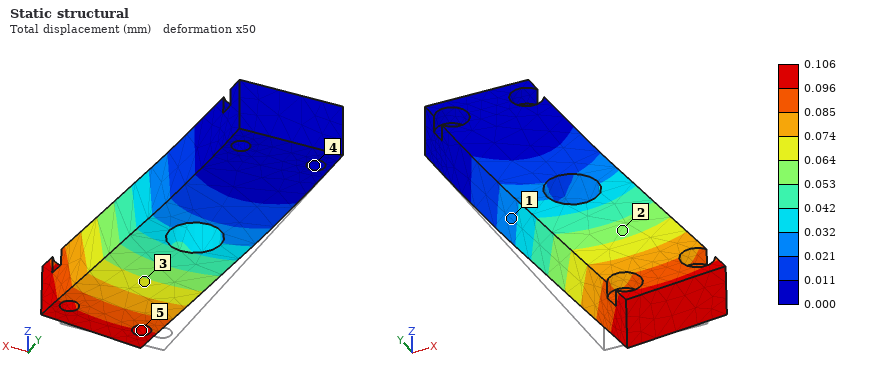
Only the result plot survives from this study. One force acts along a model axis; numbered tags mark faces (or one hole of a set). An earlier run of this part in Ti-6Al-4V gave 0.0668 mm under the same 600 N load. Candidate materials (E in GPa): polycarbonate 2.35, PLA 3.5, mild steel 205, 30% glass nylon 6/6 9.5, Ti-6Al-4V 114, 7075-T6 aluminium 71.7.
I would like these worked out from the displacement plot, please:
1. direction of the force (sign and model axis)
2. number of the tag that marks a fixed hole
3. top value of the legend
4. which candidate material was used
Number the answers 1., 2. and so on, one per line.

1. +X
2. 4
3. 0.106 mm
4. 7075-T6 aluminium
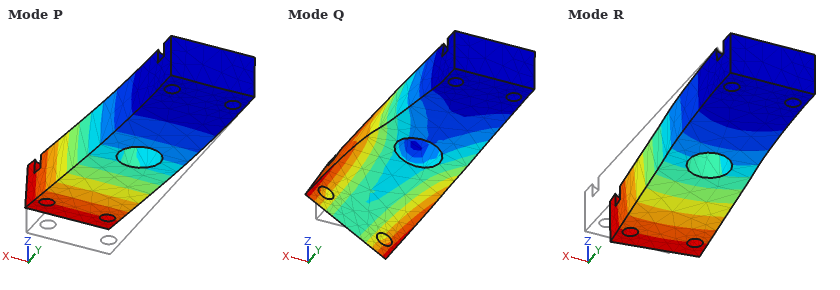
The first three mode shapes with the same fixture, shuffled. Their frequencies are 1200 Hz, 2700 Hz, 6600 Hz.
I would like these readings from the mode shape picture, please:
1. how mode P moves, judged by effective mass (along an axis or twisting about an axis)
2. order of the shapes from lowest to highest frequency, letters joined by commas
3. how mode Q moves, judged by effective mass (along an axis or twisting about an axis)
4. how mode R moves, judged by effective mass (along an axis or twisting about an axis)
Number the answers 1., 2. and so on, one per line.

1. along Z
2. P, R, Q
3. twisting about Y
4. along X
